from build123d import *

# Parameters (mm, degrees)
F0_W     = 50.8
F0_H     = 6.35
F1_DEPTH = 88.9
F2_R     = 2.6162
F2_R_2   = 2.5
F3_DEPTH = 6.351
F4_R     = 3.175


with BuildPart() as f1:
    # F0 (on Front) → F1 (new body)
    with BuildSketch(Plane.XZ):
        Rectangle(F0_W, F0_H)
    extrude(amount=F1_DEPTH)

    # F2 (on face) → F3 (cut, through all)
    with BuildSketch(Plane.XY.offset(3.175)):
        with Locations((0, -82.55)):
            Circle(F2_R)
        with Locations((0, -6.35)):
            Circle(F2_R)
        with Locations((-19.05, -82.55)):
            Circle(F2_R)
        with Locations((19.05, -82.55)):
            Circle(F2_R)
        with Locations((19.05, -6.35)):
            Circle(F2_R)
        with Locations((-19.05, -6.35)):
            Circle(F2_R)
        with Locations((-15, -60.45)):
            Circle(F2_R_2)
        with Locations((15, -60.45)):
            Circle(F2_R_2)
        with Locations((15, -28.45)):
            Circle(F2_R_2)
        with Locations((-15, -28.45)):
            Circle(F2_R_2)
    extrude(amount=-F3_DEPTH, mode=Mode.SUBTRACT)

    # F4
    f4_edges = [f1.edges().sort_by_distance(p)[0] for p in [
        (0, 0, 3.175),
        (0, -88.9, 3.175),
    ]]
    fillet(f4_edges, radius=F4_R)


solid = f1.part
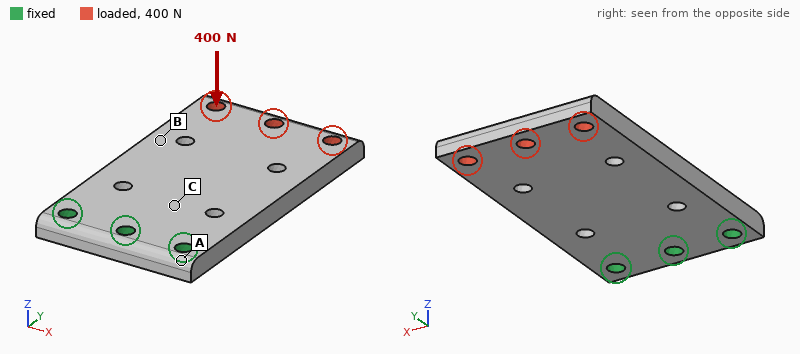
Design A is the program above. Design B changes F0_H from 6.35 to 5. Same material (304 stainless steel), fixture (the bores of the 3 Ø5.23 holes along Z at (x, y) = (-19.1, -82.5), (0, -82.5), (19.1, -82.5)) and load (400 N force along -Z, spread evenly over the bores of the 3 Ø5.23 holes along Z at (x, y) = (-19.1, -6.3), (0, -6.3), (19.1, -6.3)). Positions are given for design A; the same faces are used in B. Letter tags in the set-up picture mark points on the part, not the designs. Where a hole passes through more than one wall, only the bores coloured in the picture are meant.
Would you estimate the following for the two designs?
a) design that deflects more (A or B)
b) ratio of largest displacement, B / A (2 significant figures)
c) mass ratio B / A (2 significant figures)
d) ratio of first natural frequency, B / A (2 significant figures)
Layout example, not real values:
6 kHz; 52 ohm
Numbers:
B; 2.0; 0.79; 0.80
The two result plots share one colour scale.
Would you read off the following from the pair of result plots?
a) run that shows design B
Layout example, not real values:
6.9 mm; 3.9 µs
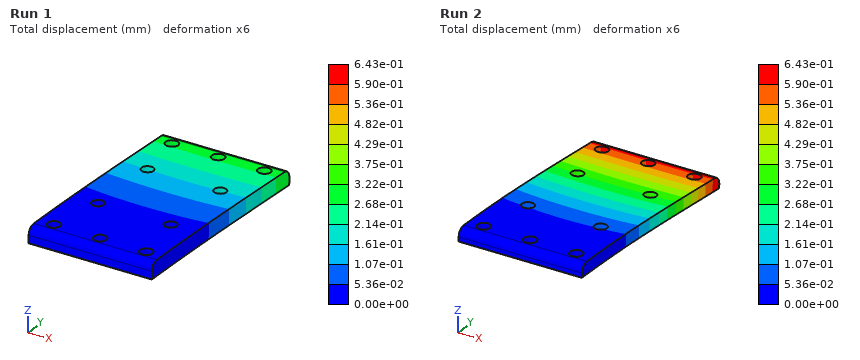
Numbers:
Run 2
